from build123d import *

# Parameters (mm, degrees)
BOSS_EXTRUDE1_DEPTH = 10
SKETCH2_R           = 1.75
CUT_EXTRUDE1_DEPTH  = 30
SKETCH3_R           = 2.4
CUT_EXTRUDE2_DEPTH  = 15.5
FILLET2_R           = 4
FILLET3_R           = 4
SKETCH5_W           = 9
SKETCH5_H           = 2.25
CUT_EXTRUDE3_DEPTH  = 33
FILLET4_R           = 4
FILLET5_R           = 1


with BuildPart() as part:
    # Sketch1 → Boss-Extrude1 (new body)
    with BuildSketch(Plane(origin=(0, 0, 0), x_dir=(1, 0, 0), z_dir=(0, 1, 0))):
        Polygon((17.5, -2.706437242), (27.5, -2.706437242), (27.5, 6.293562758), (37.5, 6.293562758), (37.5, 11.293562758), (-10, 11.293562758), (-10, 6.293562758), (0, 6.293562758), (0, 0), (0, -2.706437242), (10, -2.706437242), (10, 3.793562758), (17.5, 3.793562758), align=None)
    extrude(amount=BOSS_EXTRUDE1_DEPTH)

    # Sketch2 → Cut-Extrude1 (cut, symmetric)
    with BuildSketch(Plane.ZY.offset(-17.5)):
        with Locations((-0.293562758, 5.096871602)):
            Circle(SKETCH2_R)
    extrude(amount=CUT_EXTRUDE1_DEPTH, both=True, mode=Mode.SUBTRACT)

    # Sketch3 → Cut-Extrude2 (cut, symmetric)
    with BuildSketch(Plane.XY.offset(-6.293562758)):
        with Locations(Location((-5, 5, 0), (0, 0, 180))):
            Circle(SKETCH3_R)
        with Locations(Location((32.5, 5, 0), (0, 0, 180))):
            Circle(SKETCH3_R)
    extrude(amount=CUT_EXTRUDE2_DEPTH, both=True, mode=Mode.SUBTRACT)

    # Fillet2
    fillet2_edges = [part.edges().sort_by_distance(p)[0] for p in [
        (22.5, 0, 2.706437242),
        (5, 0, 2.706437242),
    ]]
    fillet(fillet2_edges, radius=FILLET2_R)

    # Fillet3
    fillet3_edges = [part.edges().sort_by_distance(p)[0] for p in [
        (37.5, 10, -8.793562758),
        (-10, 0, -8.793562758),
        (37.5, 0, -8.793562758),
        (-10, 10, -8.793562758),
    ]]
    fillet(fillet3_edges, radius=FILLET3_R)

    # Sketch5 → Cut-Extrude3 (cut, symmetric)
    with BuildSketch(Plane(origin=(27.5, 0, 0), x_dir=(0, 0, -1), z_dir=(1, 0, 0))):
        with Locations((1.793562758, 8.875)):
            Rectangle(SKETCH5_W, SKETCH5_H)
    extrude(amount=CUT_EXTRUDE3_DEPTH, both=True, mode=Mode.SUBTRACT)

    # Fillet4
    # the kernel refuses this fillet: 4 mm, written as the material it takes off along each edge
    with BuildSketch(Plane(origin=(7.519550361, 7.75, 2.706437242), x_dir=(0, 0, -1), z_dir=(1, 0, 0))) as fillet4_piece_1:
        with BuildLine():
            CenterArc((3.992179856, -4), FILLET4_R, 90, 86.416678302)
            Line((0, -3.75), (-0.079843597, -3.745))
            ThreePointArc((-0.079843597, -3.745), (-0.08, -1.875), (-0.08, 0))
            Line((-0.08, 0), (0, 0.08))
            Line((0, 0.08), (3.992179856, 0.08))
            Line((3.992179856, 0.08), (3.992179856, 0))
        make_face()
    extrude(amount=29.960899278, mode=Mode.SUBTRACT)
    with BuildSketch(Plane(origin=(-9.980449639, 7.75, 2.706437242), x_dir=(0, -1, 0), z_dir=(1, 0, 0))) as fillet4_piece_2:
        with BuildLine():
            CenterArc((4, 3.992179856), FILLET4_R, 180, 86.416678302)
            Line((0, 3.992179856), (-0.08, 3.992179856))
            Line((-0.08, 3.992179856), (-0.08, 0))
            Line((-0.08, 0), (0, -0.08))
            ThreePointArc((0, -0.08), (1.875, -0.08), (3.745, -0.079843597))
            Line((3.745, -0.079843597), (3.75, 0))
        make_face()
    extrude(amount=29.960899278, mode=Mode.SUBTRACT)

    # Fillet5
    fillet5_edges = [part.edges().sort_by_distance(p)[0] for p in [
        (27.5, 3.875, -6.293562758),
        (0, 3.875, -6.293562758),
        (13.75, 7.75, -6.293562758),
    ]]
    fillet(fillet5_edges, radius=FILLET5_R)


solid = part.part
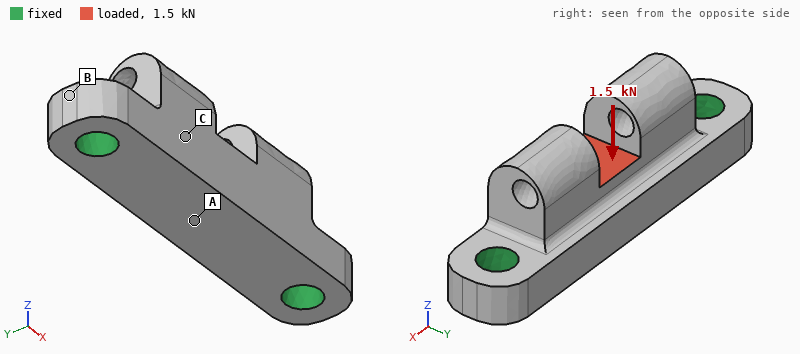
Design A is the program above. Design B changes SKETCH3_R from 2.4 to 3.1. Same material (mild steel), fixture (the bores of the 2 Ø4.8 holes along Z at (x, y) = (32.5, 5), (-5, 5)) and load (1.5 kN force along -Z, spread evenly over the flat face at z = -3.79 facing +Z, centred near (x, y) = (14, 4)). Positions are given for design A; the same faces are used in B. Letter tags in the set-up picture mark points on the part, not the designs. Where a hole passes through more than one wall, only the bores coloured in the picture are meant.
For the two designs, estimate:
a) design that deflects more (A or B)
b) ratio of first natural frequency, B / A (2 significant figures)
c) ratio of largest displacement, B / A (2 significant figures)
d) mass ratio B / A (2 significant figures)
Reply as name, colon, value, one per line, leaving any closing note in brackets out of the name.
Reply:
design that deflects more: A
ratio of first natural frequency, B / A: 1.1
ratio of largest displacement, B / A: 0.89
mass ratio B / A: 0.96
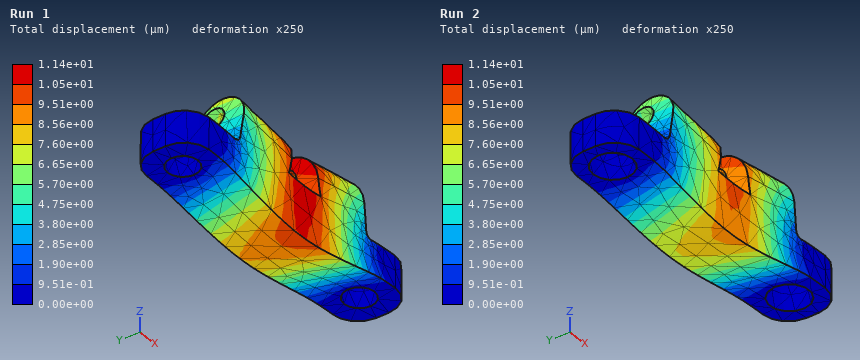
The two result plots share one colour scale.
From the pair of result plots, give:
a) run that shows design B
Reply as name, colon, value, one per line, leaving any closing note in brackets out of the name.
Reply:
run that shows design B: Run 2
